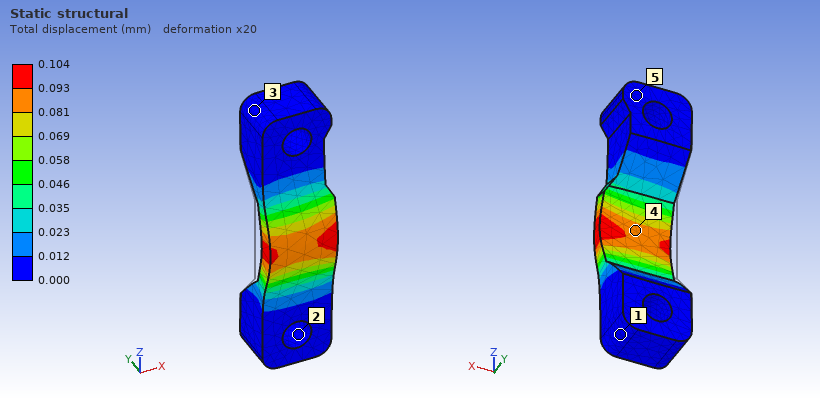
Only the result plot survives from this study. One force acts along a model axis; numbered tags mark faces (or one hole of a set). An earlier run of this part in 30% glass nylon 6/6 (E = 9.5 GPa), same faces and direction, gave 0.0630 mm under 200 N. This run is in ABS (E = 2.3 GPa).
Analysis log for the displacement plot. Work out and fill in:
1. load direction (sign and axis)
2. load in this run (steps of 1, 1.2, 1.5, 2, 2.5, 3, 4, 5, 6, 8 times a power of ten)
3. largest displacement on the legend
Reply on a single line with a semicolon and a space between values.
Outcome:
-Y; 80 N; 0.104 mm
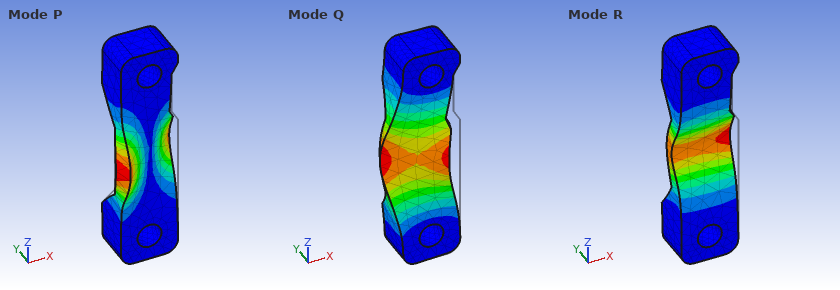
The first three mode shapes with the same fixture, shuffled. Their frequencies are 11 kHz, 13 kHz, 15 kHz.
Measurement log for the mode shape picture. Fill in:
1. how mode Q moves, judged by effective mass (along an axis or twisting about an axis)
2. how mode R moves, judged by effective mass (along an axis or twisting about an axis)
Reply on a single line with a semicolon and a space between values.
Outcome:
along X; along Y
